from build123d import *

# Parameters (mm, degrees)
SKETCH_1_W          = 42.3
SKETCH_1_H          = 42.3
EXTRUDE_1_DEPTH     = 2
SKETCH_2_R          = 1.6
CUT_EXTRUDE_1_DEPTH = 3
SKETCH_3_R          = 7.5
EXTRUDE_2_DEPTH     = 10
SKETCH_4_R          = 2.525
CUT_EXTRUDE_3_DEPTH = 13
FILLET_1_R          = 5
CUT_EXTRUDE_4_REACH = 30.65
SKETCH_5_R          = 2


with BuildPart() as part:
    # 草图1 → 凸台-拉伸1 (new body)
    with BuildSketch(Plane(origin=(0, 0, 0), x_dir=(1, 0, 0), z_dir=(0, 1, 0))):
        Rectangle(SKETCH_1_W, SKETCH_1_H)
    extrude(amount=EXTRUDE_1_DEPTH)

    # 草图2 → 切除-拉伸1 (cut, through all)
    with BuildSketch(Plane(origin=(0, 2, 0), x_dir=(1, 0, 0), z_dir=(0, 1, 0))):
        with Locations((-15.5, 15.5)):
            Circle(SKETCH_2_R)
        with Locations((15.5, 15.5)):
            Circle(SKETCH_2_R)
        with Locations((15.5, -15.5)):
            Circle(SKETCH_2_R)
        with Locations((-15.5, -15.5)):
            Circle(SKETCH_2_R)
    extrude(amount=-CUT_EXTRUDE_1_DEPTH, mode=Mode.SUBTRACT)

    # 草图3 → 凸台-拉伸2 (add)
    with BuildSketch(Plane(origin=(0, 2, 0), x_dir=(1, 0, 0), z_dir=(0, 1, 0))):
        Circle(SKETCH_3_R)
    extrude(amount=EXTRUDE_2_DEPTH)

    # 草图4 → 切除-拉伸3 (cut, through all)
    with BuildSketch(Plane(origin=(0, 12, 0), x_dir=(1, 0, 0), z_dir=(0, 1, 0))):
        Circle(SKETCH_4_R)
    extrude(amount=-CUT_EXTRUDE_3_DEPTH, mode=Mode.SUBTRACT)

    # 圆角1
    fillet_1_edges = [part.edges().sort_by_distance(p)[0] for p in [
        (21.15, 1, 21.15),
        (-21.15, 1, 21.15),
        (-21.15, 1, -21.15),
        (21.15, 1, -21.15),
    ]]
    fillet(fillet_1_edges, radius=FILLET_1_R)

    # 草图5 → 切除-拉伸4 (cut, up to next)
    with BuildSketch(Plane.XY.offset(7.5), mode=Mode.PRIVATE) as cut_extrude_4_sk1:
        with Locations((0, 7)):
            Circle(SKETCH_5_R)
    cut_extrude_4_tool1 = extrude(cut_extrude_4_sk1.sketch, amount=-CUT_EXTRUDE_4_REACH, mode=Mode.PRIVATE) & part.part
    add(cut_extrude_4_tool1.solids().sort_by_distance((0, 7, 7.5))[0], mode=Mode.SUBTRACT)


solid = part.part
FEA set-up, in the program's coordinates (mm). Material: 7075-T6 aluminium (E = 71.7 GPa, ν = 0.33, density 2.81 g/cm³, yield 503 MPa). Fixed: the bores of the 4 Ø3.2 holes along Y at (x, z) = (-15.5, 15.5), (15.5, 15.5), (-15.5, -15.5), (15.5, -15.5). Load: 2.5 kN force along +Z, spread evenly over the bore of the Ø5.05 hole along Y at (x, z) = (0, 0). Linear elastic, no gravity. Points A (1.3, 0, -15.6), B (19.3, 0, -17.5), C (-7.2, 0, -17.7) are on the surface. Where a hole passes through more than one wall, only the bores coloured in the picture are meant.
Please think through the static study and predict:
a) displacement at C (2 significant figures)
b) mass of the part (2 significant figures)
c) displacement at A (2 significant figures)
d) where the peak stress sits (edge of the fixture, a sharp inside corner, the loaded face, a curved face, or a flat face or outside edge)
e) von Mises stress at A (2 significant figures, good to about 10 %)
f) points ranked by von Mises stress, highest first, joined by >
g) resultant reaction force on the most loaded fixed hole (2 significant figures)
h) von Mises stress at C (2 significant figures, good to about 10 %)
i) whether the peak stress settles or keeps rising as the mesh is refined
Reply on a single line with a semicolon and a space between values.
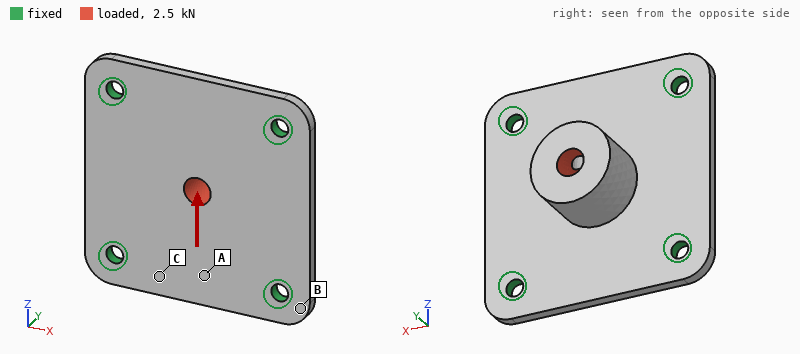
0.031 mm; 14 g; 0.058 mm; edge of the fixture; 77 MPa; A > C > B; 730 N; 40 MPa; keeps rising
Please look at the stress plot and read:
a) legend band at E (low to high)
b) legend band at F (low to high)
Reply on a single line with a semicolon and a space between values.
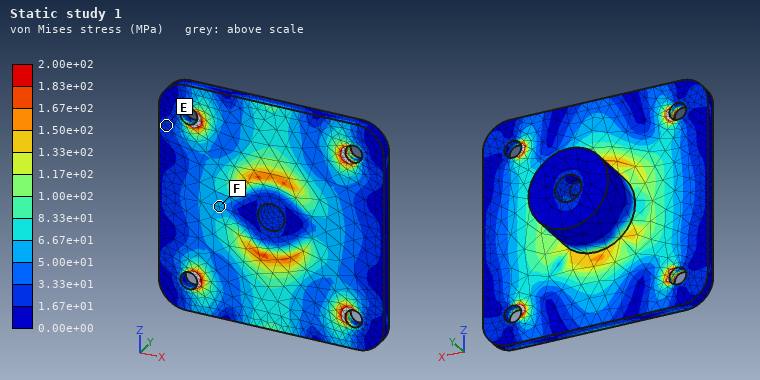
1.67e+01 to 3.33e+01 MPa; 5.00e+01 to 6.67e+01 MPa
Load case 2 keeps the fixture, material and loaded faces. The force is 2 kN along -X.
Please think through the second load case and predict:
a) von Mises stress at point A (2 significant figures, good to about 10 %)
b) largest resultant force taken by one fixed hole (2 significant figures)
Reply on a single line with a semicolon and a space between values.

32 MPa; 590 N
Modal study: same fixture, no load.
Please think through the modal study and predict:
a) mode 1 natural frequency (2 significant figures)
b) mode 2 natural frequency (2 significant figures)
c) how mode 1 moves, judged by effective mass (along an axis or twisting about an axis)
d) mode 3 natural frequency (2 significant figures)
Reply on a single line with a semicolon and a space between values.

6100 Hz; 9100 Hz; along Y; 9200 Hz
